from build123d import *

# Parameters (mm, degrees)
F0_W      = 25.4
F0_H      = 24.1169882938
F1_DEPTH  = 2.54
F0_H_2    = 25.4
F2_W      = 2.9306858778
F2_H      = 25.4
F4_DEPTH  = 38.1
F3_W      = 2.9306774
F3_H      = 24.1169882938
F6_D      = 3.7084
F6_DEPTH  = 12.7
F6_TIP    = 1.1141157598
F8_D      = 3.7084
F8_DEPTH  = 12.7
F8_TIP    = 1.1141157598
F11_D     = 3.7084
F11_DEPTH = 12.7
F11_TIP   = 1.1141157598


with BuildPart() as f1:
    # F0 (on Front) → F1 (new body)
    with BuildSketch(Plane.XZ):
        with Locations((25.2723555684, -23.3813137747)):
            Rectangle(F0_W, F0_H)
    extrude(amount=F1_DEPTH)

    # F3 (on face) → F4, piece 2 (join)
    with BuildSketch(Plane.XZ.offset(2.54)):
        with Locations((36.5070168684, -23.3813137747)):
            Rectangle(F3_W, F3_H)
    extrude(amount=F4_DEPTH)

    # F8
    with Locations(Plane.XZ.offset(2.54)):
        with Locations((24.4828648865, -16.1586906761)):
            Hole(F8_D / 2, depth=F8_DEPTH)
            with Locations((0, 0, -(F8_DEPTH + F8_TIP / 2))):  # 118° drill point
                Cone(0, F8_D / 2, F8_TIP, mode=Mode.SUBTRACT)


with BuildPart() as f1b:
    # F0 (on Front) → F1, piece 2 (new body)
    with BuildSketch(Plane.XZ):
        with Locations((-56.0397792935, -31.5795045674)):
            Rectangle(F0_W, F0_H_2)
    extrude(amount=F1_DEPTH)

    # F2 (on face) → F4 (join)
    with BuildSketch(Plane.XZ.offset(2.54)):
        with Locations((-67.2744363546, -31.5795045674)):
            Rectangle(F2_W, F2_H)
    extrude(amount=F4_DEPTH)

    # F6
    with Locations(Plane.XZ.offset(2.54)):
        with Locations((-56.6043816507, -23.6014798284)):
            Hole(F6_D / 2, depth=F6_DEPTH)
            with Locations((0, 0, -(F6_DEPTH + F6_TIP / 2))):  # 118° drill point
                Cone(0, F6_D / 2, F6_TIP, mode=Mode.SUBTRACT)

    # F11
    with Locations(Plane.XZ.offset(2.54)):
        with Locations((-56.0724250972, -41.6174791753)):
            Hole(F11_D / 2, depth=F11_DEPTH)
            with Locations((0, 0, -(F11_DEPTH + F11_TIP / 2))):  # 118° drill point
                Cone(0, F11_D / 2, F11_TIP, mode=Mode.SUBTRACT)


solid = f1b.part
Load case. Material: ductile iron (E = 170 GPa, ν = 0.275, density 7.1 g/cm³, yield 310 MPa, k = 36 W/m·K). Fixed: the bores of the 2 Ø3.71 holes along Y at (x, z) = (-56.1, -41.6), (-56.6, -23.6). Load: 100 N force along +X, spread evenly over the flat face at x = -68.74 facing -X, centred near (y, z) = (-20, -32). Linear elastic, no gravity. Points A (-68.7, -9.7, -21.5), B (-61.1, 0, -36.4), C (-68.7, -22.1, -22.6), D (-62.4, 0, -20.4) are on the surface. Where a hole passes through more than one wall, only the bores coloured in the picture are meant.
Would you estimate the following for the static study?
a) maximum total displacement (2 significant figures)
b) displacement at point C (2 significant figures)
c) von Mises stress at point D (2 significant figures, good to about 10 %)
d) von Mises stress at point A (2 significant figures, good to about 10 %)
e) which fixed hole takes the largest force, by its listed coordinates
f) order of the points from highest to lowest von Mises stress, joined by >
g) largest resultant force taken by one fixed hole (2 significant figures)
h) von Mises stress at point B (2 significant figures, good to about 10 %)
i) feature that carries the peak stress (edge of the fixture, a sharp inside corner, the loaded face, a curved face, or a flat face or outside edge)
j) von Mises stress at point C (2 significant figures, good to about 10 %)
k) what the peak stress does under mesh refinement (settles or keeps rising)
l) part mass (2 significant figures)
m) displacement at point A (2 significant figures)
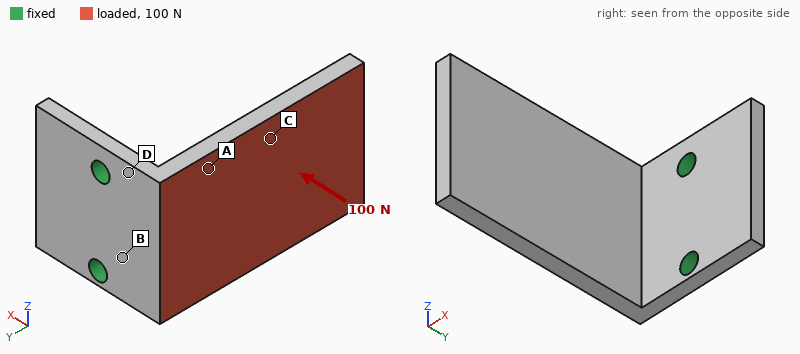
0.20 mm
0.094 mm
72 MPa
33 MPa
(-56.6, -23.6)
D > B > A > C
58 N
55 MPa
edge of the fixture
12 MPa
keeps rising
31 g
0.038 mm
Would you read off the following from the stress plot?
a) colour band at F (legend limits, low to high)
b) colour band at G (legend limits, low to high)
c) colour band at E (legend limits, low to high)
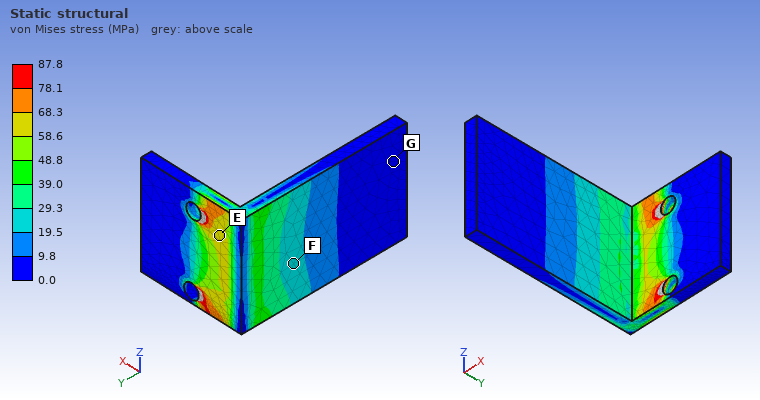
19.5 to 29.3 MPa
0.0 to 9.8 MPa
58.6 to 68.3 MPa
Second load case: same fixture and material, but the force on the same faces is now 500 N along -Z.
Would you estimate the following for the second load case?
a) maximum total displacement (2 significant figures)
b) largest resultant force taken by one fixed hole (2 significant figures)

0.13 mm
650 N
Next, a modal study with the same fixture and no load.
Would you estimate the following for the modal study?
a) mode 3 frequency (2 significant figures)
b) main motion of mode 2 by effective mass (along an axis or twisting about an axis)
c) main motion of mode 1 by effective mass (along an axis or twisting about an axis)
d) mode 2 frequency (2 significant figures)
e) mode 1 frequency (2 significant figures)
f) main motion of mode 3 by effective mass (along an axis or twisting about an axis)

4900 Hz
along Z
along X
2500 Hz
950 Hz
twisting about Y
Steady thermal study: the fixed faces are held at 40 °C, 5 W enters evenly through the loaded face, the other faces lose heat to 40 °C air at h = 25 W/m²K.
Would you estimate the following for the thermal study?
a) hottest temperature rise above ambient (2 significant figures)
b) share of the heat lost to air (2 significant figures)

42 K
25 %
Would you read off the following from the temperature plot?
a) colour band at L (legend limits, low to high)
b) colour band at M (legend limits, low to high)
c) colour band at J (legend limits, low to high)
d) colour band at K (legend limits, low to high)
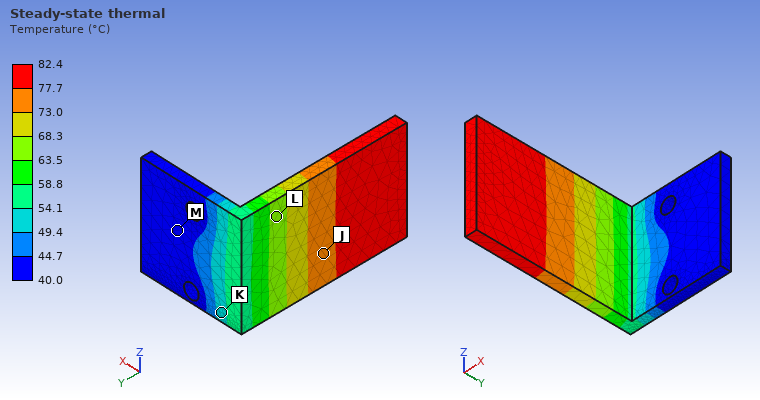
63.5 to 68.3 °C
40.0 to 44.7 °C
73.0 to 77.7 °C
49.4 to 54.1 °C
